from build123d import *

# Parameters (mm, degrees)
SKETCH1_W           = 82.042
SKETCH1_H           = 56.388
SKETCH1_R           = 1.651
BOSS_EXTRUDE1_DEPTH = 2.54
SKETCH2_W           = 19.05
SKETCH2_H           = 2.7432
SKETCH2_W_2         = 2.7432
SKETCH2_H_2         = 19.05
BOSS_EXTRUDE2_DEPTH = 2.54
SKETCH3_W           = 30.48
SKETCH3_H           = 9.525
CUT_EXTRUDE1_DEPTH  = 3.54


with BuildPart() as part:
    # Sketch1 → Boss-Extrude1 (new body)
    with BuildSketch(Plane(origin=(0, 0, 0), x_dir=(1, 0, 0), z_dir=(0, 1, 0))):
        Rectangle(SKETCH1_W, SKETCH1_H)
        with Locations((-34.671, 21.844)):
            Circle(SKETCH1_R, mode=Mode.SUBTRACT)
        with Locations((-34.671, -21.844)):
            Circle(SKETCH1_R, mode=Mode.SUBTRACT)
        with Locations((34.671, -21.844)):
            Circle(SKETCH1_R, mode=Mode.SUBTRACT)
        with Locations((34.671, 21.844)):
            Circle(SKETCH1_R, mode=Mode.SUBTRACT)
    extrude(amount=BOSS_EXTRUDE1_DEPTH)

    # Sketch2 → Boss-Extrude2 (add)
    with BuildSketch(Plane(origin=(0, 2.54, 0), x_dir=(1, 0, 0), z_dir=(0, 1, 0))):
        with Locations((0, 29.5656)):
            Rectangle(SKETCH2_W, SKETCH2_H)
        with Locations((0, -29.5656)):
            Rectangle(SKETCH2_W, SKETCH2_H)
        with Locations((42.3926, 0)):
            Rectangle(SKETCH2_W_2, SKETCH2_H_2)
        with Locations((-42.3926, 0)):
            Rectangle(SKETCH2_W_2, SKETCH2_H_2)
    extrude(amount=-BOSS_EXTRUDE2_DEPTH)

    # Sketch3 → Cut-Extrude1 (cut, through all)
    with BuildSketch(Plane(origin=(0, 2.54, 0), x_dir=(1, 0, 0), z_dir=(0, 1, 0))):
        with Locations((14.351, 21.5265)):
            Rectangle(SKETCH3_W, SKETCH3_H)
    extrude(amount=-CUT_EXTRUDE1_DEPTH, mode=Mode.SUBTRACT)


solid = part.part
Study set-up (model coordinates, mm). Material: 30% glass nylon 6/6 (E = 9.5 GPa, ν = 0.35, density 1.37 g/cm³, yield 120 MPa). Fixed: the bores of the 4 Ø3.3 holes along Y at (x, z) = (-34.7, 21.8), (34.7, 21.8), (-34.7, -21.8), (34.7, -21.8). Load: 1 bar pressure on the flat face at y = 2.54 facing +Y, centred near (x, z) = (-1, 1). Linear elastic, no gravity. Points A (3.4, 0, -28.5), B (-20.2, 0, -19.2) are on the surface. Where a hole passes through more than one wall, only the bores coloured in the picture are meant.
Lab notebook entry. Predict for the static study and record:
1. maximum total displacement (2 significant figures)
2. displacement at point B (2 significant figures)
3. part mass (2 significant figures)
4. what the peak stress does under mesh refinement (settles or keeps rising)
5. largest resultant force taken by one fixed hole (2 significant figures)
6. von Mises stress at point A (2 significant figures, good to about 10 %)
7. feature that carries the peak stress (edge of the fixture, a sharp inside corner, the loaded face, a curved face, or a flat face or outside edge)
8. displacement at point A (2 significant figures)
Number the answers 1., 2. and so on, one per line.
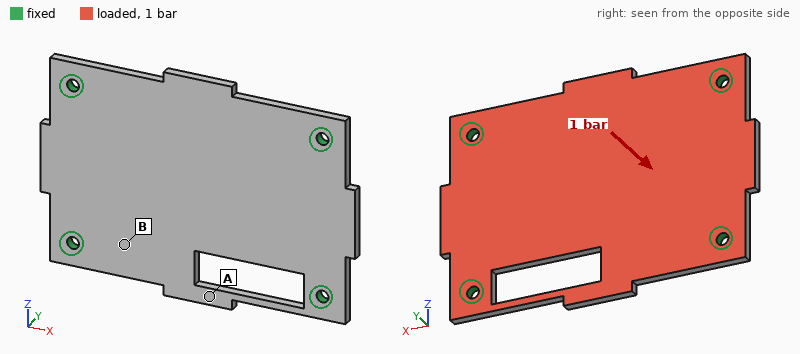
1. 0.69 mm
2. 0.29 mm
3. 16 g
4. keeps rising
5. 120 N
6. 25 MPa
7. edge of the fixture
8. 0.66 mm
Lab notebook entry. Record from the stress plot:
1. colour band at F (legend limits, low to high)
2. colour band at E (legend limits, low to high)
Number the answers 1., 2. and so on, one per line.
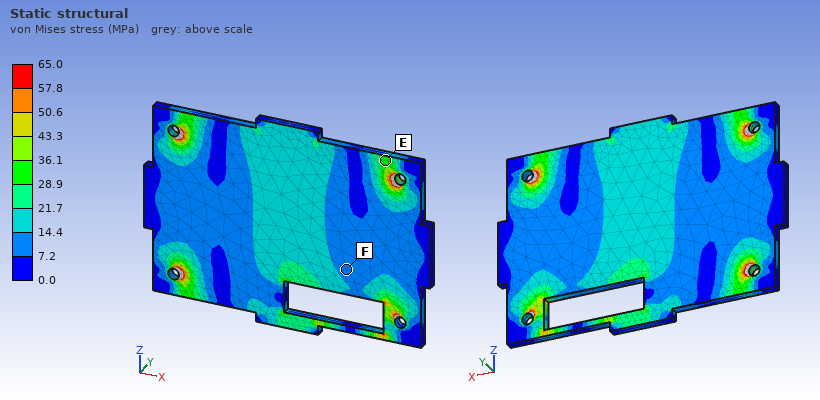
1. 7.2 to 14.4 MPa
2. 28.9 to 36.1 MPa
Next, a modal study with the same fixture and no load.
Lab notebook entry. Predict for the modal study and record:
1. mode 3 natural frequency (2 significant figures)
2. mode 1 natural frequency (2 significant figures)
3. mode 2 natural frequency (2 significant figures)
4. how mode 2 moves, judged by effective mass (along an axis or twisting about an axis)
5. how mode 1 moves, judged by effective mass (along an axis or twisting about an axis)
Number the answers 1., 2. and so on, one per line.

1. 2600 Hz
2. 1200 Hz
3. 1700 Hz
4. twisting about X
5. along Y
